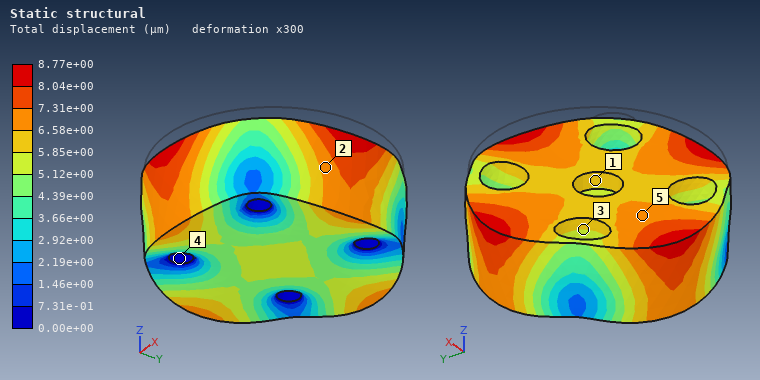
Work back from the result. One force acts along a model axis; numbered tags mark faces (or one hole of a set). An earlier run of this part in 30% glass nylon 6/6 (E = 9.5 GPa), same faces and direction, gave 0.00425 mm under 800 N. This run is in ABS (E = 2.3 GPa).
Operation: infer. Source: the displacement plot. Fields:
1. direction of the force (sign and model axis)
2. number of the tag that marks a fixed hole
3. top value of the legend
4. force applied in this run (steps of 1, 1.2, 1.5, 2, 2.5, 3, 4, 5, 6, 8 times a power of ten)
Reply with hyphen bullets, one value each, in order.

- -Z
- 4
- 8.77e+00 µm
- 400 N
